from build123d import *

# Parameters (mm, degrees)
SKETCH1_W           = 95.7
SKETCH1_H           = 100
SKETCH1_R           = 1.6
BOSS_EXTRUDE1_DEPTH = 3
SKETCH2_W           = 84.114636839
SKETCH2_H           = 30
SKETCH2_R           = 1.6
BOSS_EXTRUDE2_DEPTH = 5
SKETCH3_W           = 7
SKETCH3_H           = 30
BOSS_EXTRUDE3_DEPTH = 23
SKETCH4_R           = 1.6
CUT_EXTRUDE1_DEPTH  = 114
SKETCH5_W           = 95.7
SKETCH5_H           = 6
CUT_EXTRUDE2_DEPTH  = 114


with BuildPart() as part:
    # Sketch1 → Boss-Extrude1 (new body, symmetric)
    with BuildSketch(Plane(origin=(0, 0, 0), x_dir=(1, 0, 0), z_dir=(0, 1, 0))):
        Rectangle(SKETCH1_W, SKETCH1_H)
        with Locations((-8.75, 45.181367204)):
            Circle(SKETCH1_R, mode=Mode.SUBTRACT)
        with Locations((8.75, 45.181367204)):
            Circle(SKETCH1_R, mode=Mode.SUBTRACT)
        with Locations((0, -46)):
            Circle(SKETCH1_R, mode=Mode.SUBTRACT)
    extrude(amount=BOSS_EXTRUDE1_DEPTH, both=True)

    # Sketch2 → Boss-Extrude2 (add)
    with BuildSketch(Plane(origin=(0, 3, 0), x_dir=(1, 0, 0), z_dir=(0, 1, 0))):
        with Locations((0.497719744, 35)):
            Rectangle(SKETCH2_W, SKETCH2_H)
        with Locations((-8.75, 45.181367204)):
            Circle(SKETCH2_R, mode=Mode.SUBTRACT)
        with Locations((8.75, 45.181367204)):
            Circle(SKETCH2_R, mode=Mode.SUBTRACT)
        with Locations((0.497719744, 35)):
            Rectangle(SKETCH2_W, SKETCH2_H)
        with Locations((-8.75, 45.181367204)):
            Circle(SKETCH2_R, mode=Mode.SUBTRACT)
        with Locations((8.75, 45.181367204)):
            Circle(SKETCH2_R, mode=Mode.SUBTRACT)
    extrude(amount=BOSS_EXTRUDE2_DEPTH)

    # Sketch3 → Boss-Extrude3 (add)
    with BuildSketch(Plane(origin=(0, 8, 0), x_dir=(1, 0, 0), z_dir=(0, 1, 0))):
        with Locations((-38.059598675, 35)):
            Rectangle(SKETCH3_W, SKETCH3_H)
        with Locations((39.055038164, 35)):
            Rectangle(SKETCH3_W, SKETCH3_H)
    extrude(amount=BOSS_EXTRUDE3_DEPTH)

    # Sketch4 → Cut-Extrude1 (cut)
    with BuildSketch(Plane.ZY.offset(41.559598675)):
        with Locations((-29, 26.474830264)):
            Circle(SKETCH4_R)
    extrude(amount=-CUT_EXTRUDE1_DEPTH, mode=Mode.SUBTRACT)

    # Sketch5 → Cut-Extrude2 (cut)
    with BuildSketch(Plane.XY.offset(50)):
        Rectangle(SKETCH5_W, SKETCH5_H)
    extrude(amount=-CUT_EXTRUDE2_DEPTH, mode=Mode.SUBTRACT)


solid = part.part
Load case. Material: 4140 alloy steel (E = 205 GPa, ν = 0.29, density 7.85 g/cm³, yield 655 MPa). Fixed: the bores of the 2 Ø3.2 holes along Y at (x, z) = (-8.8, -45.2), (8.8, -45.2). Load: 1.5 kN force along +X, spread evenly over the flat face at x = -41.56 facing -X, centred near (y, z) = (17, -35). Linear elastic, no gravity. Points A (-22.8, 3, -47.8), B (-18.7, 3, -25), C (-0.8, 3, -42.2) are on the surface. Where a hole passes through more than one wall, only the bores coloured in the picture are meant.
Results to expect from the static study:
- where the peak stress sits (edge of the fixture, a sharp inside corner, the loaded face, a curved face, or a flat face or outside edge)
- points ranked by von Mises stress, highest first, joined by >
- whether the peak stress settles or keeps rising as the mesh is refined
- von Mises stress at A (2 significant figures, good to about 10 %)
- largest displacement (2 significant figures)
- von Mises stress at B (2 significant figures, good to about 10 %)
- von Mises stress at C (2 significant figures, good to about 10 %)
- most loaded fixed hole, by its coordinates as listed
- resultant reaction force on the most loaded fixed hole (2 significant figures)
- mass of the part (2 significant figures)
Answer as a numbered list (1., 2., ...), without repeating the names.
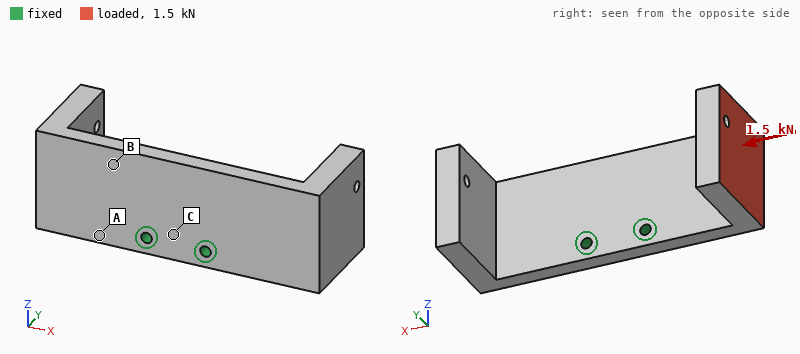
1. edge of the fixture
2. A > B > C
3. keeps rising
4. 140 MPa
5. 0.29 mm
6. 110 MPa
7. 21 MPa
8. (-8.8, -45.2)
9. 1.3 kN
10. 170 g
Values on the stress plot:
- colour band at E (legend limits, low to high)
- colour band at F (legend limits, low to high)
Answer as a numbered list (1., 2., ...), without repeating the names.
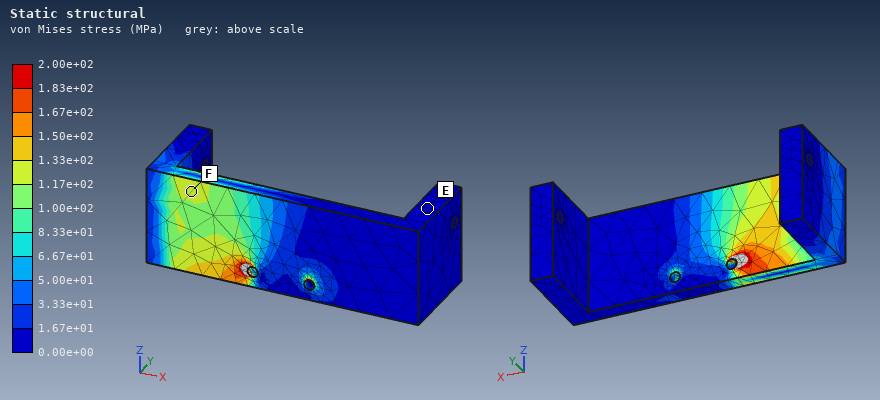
1. 0.00e+00 to 1.67e+01 MPa
2. 1.17e+02 to 1.33e+02 MPa
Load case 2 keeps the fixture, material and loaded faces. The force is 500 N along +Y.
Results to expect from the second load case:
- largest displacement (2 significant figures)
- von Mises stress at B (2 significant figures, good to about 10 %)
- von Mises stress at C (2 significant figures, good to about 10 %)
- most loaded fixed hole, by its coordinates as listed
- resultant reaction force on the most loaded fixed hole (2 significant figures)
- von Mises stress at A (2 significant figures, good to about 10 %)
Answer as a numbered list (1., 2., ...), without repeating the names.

1. 0.20 mm
2. 76 MPa
3. 29 MPa
4. (-8.8, -45.2)
5. 920 N
6. 88 MPa
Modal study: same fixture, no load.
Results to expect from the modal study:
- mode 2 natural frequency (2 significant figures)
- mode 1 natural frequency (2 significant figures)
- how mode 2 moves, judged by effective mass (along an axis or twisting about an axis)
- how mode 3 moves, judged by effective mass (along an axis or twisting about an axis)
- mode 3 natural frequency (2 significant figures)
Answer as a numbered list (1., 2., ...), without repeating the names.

1. 1400 Hz
2. 1300 Hz
3. along Y
4. along Z
5. 2200 Hz
